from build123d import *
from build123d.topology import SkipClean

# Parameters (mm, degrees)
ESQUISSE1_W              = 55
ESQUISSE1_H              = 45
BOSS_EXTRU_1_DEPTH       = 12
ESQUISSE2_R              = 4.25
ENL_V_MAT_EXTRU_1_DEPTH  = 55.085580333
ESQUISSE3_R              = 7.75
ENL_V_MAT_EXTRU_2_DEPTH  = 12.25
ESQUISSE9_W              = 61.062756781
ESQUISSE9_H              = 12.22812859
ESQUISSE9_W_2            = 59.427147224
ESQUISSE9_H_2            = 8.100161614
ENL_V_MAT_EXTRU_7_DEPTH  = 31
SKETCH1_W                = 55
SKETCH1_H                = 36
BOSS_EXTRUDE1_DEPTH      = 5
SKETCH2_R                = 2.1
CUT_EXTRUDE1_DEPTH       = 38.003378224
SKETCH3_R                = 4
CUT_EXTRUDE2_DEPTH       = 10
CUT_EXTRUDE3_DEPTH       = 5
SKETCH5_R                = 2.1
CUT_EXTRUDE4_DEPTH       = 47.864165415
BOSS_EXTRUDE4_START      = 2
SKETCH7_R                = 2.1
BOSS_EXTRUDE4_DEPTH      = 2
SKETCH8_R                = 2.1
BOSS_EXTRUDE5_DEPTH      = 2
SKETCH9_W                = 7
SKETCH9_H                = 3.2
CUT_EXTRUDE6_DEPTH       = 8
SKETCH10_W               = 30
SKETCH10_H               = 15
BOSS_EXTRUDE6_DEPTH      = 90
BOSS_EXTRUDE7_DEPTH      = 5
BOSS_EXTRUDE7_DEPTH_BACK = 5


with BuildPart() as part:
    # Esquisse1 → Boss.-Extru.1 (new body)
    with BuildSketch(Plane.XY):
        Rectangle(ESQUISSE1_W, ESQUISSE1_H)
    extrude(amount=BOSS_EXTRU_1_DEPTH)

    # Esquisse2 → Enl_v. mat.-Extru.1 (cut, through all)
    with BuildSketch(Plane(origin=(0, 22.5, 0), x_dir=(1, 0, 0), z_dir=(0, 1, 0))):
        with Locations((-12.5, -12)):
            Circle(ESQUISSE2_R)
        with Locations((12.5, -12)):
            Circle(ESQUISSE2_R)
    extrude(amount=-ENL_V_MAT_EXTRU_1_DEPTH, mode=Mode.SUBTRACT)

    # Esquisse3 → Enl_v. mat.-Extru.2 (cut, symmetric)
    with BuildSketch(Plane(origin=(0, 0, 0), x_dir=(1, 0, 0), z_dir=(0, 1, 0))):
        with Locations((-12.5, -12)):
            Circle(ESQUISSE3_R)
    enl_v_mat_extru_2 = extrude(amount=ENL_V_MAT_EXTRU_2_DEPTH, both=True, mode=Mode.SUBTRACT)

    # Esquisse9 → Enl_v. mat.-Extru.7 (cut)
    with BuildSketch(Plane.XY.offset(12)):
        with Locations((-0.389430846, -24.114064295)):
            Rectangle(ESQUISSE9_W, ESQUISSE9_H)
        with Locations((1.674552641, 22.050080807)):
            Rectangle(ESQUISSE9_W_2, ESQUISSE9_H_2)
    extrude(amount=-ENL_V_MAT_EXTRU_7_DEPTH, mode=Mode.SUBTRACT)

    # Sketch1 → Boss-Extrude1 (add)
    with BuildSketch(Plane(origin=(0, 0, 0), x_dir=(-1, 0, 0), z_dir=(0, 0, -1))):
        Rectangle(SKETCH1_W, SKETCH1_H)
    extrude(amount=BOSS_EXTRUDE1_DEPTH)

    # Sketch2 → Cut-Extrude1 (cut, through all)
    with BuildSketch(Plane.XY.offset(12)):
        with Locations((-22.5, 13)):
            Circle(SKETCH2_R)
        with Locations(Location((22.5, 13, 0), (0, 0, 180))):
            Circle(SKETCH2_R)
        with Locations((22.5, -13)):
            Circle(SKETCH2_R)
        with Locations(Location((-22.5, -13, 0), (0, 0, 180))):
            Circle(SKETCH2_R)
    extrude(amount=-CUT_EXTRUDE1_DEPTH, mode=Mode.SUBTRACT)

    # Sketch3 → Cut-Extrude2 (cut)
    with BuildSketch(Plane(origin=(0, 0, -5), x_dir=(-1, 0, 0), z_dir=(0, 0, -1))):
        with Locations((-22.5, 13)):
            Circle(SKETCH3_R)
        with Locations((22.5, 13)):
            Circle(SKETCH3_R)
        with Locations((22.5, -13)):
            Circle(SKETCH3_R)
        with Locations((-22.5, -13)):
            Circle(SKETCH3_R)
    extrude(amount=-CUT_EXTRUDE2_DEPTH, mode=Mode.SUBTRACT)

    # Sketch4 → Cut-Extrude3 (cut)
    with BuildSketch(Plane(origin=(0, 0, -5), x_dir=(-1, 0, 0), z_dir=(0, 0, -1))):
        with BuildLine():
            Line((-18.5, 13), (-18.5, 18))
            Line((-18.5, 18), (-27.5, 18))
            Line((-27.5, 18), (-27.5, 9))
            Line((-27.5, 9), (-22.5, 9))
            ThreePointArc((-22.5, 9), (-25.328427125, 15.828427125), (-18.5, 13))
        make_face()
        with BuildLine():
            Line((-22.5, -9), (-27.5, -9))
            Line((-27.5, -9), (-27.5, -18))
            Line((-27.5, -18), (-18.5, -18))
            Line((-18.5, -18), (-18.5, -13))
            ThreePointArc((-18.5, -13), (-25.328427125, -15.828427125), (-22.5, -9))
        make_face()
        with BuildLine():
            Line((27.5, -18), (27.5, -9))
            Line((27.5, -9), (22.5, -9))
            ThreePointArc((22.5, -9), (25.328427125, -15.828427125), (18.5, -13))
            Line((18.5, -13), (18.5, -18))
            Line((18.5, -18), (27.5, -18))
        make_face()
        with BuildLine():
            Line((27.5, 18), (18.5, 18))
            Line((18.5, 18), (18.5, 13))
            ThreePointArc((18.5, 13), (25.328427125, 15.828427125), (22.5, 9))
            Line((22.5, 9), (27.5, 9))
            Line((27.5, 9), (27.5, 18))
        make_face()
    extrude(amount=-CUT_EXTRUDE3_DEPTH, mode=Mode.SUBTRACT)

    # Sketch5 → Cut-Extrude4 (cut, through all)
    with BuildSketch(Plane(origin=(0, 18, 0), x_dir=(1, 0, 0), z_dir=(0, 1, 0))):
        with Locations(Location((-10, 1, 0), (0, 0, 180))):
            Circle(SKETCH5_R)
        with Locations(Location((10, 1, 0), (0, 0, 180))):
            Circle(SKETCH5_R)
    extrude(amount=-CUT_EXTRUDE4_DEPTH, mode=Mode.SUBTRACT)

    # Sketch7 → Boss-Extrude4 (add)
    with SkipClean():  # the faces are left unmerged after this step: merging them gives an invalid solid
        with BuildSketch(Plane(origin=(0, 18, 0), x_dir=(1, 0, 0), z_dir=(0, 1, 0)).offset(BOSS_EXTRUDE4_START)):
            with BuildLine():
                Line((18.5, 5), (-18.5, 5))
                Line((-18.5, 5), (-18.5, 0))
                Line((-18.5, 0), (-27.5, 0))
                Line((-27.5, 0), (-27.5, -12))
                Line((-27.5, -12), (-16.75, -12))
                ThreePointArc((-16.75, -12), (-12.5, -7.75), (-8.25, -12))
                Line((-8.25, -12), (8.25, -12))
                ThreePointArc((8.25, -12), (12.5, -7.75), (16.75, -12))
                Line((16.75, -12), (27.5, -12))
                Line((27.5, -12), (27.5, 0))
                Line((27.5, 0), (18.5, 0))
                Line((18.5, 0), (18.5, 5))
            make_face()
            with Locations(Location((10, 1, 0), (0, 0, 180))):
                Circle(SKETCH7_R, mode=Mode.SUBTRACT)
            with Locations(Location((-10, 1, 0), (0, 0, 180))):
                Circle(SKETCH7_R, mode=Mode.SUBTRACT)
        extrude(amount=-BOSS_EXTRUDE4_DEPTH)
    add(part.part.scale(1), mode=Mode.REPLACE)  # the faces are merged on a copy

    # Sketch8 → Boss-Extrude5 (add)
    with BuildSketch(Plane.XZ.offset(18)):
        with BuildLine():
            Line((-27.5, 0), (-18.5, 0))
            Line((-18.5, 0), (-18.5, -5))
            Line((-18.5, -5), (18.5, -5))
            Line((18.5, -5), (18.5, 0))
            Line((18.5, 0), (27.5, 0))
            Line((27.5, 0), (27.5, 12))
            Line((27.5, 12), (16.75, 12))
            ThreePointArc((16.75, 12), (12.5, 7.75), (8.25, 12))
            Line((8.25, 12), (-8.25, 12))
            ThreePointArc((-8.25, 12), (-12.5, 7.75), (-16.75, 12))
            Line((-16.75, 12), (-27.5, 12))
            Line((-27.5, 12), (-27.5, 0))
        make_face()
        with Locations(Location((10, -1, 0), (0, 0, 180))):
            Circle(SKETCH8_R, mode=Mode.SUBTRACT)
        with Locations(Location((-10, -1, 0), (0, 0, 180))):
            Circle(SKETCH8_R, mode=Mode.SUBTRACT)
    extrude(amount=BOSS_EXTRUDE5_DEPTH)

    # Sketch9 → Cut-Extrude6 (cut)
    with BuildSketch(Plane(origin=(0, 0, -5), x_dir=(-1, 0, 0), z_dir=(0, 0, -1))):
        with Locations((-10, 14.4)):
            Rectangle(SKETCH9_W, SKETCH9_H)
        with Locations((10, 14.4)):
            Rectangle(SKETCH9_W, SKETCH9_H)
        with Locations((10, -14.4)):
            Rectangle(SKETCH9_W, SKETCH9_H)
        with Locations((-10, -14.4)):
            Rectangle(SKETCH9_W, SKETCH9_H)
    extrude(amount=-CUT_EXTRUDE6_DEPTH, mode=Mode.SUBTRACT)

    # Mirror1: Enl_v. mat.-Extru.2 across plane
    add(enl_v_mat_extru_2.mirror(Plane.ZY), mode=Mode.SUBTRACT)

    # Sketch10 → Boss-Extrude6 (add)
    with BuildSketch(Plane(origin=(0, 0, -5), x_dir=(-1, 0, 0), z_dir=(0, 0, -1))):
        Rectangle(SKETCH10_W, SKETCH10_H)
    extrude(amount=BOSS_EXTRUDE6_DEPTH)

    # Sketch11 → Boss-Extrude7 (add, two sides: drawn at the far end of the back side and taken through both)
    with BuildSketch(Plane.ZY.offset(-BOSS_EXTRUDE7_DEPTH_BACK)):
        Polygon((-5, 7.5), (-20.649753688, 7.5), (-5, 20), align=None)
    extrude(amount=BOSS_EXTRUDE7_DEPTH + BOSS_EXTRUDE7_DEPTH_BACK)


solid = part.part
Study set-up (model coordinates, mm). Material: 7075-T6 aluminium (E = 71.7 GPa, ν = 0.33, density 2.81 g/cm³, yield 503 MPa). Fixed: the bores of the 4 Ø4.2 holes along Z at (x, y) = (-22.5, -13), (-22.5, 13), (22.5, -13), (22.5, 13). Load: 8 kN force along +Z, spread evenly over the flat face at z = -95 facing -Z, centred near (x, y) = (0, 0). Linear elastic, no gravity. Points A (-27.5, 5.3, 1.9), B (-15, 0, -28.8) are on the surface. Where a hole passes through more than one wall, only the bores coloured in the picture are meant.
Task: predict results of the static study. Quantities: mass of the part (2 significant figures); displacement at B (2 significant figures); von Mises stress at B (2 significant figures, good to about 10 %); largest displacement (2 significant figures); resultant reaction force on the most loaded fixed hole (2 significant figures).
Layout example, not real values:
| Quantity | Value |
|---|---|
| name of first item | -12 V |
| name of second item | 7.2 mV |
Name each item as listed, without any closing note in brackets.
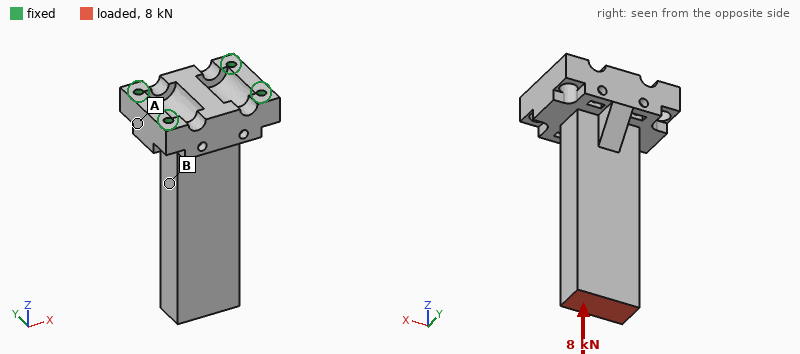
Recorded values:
| Quantity | Value |
|---|---|
| mass of the part | 190 g |
| displacement at B | 19 µm |
| von Mises stress at B | 17 MPa |
| largest displacement | 38 µm |
| resultant reaction force on the most loaded fixed hole | 2.4 kN |
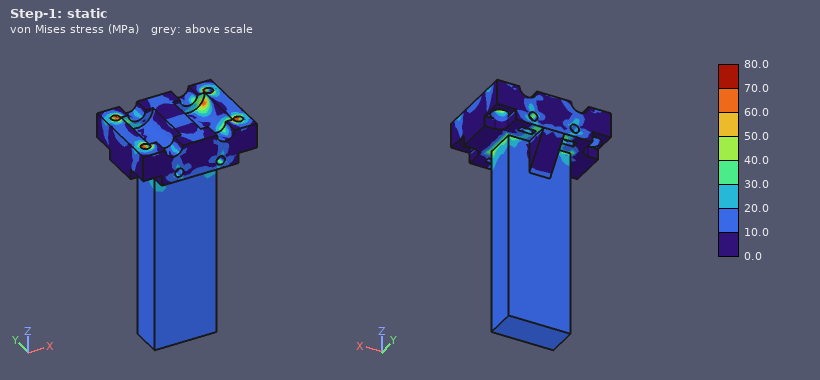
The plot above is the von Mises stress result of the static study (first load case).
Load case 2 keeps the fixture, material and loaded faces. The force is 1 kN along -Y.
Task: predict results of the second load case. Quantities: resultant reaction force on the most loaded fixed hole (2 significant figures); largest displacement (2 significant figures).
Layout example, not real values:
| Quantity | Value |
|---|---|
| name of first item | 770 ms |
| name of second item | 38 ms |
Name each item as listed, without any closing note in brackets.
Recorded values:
| Quantity | Value |
|---|---|
| resultant reaction force on the most loaded fixed hole | 2.1 kN |
| largest displacement | 0.48 mm |
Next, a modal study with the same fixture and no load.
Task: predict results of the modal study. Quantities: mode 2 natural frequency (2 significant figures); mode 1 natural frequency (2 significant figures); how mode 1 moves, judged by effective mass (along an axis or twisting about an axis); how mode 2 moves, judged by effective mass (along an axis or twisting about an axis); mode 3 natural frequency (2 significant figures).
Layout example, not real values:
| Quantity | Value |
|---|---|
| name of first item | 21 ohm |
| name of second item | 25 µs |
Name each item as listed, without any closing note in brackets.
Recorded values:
| Quantity | Value |
|---|---|
| mode 2 natural frequency | 2200 Hz |
| mode 1 natural frequency | 1300 Hz |
| how mode 1 moves, judged by effective mass | along Y |
| how mode 2 moves, judged by effective mass | along X |
| mode 3 natural frequency | 6400 Hz |
